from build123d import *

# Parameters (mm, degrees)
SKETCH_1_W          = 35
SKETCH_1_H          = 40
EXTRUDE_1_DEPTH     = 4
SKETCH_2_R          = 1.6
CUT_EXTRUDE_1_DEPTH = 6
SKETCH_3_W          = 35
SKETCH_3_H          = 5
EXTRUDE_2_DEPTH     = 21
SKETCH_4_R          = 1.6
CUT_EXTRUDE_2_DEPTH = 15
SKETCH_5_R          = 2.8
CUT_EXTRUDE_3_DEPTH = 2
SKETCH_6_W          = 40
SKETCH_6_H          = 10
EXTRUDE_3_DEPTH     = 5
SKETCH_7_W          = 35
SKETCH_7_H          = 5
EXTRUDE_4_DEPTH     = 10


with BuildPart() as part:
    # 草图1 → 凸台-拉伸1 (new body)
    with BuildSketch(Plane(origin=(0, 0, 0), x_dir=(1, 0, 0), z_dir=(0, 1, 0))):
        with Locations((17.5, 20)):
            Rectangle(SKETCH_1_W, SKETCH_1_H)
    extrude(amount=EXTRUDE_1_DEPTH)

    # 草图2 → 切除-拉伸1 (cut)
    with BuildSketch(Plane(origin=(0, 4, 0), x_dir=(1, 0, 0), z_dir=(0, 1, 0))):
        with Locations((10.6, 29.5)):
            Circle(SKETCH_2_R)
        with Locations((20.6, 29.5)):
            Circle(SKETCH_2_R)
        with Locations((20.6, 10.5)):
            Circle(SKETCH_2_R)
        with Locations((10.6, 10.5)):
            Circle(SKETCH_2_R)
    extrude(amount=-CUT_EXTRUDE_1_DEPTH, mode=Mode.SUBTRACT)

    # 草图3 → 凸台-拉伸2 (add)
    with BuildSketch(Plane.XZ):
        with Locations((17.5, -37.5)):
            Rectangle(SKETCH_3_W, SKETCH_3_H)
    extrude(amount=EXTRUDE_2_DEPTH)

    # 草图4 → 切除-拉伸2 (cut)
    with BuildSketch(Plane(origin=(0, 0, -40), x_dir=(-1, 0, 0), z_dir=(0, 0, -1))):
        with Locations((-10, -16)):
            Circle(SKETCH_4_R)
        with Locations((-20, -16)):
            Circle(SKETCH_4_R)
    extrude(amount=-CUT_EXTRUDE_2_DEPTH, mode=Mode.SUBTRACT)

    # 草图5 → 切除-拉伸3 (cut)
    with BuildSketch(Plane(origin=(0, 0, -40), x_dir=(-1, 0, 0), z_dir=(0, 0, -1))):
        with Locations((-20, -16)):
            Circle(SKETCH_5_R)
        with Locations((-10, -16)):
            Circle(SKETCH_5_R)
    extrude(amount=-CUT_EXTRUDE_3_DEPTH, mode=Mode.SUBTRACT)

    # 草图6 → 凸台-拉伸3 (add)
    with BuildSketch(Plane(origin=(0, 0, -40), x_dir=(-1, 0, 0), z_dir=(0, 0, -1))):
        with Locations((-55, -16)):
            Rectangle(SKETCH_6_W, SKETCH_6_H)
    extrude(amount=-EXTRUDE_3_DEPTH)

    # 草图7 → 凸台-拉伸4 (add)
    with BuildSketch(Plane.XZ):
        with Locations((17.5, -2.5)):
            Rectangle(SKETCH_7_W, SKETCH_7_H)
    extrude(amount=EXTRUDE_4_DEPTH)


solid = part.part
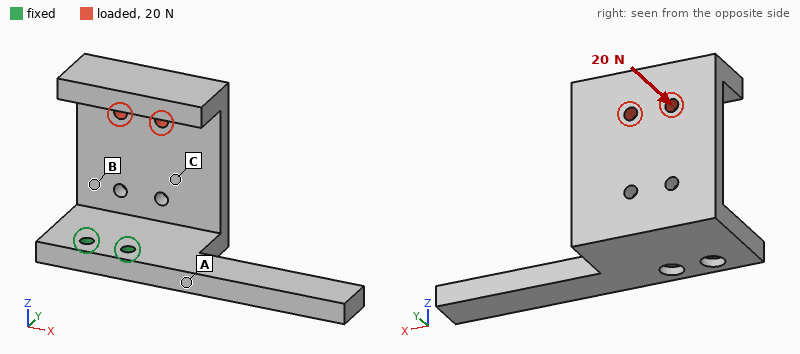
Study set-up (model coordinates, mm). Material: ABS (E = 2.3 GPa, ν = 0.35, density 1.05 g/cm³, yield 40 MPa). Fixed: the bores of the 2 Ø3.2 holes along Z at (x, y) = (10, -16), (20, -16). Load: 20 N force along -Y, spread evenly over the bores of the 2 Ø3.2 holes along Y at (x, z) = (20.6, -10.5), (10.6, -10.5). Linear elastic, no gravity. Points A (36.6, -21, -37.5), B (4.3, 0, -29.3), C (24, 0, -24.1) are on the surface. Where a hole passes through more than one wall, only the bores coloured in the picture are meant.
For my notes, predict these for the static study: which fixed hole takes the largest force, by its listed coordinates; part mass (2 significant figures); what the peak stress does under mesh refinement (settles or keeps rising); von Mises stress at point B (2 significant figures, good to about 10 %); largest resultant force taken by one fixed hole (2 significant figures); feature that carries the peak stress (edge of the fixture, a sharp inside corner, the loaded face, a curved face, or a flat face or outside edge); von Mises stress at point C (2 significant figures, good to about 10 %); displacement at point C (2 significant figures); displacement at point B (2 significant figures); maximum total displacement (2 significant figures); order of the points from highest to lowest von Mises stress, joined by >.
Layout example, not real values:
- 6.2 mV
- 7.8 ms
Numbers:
- (20, -16)
- 13 g
- keeps rising
- 4.3 MPa
- 14 N
- edge of the fixture
- 2.8 MPa
- 0.31 mm
- 0.20 mm
- 1.1 mm
- B > C > A
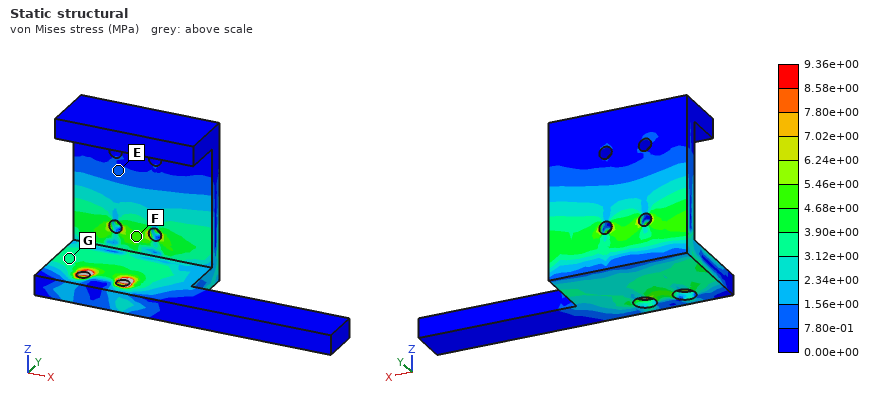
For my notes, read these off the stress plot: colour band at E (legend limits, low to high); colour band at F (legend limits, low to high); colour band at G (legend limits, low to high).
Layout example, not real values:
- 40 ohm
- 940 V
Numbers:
- 7.80e-01 to 1.56e+00 MPa
- 4.68e+00 to 5.46e+00 MPa
- 3.12e+00 to 3.90e+00 MPa
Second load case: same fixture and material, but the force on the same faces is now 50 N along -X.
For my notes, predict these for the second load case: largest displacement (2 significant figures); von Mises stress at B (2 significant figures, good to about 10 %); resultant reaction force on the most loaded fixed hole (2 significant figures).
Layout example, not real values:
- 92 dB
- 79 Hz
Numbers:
- 0.94 mm
- 4.2 MPa
- 110 N
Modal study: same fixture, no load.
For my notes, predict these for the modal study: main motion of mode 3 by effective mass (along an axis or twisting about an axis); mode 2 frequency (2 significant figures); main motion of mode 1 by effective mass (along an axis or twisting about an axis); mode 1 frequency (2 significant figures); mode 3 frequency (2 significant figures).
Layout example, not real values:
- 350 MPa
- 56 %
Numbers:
- along X
- 410 Hz
- along Y
- 310 Hz
- 580 Hz
